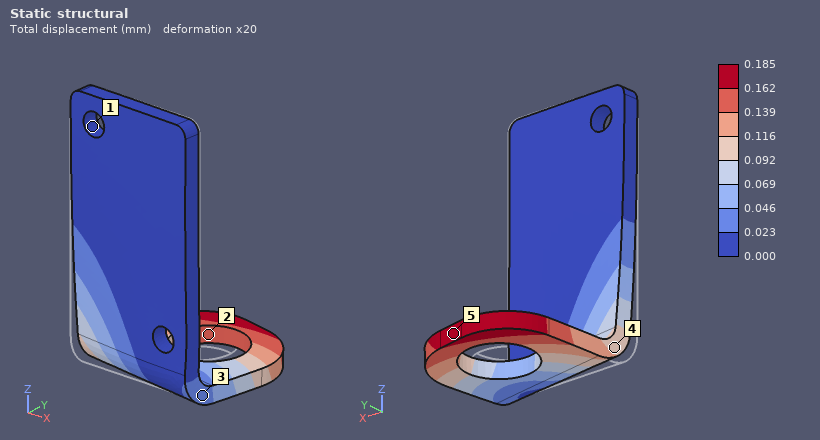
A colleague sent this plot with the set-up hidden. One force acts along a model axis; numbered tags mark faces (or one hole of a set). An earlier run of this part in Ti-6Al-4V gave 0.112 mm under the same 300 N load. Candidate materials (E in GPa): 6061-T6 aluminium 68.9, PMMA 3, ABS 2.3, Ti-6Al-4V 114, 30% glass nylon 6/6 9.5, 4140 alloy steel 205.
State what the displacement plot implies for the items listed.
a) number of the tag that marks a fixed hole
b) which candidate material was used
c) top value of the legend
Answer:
1
6061-T6 aluminium
0.185 mm
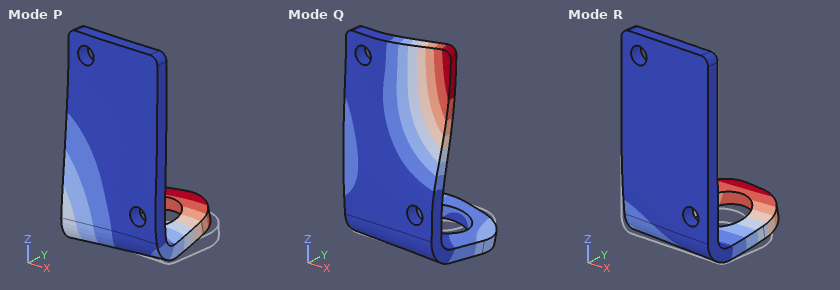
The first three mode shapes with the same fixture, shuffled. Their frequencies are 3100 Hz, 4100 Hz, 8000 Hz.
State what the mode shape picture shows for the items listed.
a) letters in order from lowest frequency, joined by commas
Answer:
R, P, Q
